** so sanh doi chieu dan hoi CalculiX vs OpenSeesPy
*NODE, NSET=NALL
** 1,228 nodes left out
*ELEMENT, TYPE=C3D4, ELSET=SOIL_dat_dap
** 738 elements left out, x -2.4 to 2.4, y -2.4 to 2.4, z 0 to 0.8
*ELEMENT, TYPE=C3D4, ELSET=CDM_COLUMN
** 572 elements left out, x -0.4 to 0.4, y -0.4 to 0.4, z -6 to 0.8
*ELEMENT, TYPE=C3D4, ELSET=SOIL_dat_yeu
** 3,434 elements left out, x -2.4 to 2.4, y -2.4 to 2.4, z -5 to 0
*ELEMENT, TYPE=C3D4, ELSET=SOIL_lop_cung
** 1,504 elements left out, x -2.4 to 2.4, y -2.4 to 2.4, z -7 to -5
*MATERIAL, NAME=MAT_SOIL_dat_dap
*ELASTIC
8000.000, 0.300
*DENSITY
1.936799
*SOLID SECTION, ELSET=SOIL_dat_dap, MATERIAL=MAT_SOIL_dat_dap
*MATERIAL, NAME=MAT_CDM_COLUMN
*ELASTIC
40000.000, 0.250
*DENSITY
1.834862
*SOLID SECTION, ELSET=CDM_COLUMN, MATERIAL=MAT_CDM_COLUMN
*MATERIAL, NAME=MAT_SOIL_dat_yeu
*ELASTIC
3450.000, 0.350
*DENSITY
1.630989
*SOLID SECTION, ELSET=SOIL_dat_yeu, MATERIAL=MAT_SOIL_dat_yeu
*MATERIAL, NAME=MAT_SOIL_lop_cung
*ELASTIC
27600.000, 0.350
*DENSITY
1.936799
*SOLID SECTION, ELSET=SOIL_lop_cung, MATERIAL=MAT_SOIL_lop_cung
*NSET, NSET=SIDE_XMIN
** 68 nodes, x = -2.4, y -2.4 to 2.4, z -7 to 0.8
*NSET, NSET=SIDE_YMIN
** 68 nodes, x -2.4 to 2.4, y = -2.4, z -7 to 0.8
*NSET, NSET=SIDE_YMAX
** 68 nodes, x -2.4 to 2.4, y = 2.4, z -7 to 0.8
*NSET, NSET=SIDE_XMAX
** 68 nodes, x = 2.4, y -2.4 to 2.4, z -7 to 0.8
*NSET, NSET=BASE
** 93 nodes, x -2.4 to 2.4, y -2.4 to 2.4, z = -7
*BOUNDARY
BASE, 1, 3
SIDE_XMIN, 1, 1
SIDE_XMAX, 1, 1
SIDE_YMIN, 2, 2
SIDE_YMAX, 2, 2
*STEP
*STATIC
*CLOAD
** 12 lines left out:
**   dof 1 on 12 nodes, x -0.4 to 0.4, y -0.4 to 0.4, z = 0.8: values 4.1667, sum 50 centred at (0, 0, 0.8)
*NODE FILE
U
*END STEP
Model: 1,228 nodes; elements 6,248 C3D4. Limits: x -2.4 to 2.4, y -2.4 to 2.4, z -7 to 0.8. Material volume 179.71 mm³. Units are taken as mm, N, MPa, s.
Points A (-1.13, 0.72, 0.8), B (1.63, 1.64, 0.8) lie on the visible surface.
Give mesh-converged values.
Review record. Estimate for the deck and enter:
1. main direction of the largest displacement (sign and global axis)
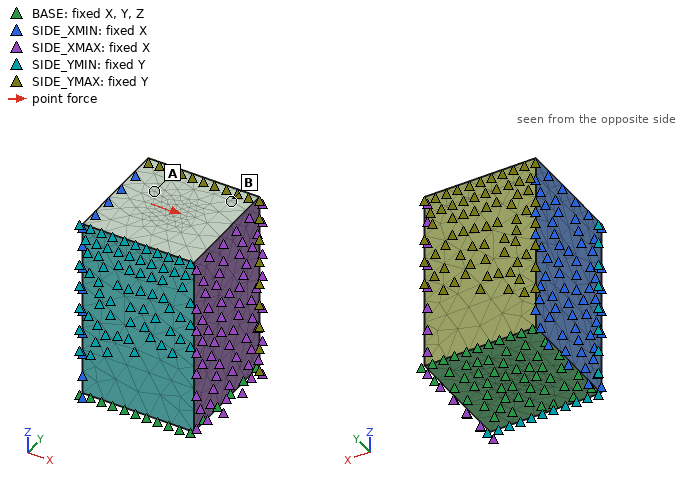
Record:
+X
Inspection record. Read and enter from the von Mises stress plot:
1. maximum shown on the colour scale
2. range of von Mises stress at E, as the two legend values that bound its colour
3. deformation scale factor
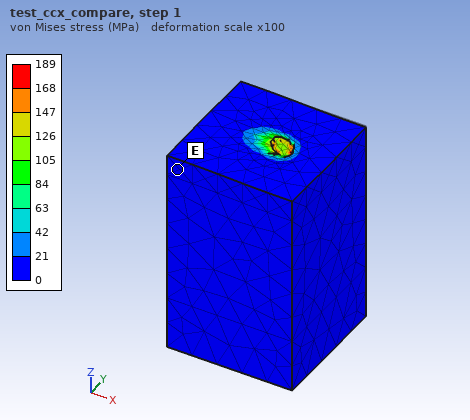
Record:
189 MPa
0 to 21 MPa
100
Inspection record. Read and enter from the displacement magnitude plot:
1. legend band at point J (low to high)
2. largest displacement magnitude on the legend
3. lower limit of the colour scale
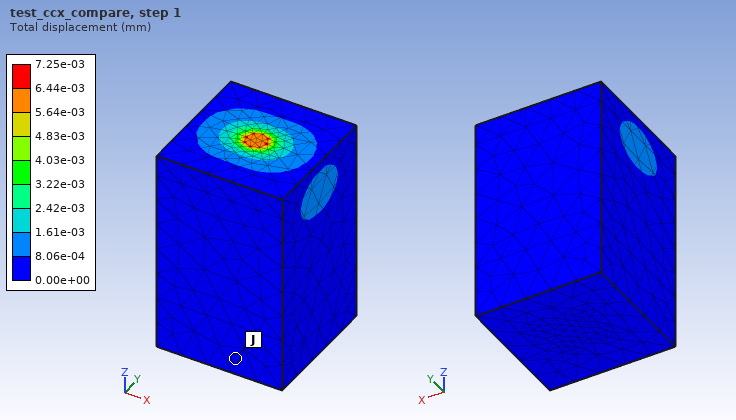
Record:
0.00e+00 to 8.06e-04 mm
7.25e-03 mm
0.00e+00 mm
